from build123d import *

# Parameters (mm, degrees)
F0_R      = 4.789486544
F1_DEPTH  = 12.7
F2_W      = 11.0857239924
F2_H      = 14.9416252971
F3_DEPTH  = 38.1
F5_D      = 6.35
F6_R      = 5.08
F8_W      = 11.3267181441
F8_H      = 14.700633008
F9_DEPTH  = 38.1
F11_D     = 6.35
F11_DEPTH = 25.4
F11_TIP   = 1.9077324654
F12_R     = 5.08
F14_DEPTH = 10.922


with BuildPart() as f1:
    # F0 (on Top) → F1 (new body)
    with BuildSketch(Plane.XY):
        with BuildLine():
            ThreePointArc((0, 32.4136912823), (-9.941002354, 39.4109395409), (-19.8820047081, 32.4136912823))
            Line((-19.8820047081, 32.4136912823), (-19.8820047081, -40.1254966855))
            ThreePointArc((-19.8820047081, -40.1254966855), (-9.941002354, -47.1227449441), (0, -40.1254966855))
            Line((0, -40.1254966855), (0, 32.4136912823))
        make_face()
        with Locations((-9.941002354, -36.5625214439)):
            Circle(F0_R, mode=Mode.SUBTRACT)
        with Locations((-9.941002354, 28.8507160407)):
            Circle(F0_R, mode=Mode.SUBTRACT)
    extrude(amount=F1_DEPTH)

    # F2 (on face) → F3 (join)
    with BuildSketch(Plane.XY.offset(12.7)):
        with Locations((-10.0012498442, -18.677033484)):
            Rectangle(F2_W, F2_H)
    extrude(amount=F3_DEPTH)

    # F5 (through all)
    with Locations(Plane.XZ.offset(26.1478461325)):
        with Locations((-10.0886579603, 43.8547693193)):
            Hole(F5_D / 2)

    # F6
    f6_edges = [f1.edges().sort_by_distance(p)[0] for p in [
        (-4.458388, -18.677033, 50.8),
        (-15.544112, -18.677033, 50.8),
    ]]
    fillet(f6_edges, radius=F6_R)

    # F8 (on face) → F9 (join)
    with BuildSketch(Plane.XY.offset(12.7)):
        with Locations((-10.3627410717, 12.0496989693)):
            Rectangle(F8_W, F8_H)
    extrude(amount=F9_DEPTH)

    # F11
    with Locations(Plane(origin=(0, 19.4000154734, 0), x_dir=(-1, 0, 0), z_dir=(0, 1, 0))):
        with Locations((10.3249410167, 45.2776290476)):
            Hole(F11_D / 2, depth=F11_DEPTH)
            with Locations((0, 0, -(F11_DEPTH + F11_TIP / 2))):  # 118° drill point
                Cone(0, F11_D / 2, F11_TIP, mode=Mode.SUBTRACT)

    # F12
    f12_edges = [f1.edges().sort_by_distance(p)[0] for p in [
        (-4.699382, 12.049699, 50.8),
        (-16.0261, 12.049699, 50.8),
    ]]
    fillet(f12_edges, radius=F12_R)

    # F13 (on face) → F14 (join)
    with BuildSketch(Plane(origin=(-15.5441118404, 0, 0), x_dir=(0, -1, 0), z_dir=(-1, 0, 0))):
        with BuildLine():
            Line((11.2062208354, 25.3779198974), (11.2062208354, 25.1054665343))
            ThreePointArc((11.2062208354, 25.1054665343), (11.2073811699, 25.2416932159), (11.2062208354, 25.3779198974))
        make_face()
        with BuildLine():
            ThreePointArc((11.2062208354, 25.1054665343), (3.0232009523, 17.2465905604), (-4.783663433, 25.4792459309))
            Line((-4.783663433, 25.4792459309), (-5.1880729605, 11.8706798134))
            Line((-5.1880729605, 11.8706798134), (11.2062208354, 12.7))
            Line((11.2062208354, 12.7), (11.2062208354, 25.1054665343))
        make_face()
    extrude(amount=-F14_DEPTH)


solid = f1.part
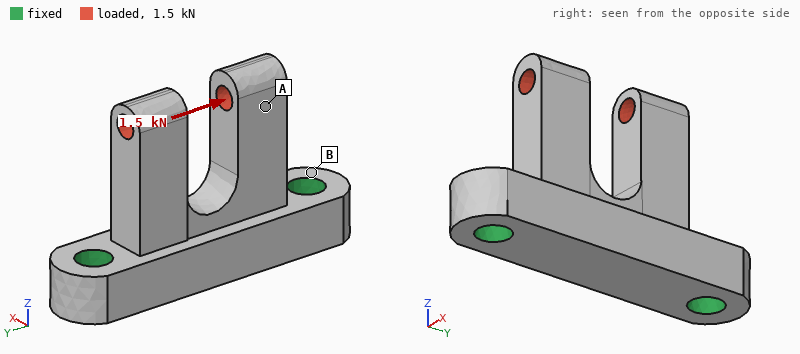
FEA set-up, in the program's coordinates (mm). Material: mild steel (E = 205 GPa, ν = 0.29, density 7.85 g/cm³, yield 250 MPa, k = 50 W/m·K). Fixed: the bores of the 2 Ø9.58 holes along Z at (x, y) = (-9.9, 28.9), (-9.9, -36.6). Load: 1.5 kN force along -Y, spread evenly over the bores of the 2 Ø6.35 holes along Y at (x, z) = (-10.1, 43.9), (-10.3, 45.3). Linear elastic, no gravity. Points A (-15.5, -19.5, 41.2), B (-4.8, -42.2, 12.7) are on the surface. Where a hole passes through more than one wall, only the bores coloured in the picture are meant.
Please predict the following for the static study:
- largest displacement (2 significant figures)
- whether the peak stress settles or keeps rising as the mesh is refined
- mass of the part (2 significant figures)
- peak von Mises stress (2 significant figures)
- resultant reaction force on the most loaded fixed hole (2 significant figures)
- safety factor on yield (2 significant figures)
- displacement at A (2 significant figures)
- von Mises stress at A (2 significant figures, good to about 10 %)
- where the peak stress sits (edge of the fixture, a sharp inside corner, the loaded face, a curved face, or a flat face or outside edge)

19 µm
settles
250 g
60 MPa
1.3 kN
4.2
11 µm
12 MPa
a curved face
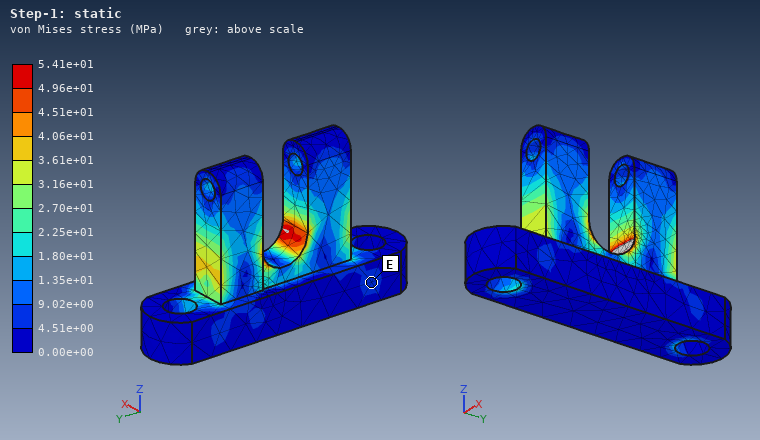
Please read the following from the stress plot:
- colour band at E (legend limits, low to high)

4.51e+00 to 9.02e+00 MPa
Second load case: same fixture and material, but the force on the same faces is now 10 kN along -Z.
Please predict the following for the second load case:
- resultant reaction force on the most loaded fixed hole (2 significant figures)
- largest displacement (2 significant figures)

5.2 kN
16 µm
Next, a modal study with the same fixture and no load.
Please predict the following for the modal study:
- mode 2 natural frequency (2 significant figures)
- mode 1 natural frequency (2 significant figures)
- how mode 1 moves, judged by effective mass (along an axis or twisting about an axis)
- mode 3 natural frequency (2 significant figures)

6000 Hz
4700 Hz
along X
7900 Hz
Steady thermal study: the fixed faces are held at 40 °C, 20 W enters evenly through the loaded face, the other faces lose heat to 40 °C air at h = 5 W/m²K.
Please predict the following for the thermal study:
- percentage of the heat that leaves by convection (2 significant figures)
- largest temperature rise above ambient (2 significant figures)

4.0 %
54 K
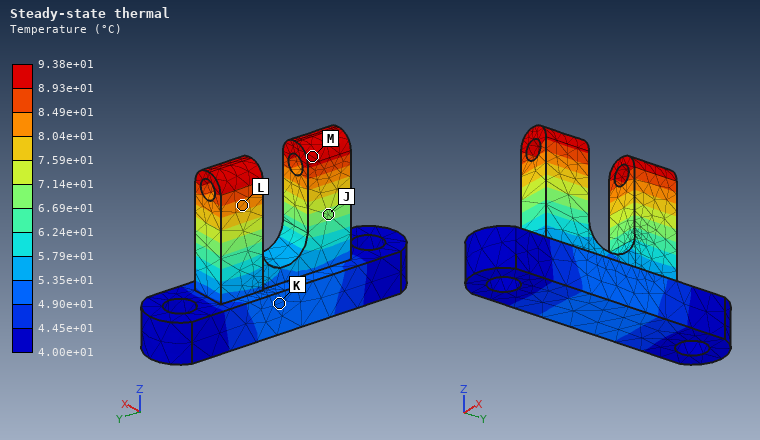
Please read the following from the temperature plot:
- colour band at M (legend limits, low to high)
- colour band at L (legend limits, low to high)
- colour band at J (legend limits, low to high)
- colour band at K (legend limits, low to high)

8.93e+01 to 9.38e+01 °C
8.04e+01 to 8.49e+01 °C
6.69e+01 to 7.14e+01 °C
4.90e+01 to 5.35e+01 °C
